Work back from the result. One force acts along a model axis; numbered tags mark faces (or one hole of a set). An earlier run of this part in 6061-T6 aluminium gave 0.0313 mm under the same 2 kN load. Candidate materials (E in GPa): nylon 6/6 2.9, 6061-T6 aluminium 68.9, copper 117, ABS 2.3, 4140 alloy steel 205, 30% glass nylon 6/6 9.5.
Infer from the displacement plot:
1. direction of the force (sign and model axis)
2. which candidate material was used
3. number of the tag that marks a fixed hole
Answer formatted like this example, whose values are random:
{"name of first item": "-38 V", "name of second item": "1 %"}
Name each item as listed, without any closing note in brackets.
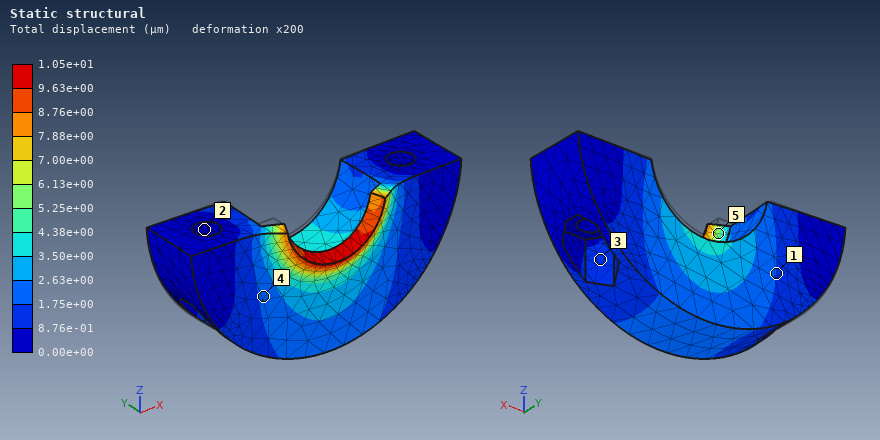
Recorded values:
{"direction of the force": "-Y", "which candidate material was used": "4140 alloy steel", "number of the tag that marks a fixed hole": "2"}
